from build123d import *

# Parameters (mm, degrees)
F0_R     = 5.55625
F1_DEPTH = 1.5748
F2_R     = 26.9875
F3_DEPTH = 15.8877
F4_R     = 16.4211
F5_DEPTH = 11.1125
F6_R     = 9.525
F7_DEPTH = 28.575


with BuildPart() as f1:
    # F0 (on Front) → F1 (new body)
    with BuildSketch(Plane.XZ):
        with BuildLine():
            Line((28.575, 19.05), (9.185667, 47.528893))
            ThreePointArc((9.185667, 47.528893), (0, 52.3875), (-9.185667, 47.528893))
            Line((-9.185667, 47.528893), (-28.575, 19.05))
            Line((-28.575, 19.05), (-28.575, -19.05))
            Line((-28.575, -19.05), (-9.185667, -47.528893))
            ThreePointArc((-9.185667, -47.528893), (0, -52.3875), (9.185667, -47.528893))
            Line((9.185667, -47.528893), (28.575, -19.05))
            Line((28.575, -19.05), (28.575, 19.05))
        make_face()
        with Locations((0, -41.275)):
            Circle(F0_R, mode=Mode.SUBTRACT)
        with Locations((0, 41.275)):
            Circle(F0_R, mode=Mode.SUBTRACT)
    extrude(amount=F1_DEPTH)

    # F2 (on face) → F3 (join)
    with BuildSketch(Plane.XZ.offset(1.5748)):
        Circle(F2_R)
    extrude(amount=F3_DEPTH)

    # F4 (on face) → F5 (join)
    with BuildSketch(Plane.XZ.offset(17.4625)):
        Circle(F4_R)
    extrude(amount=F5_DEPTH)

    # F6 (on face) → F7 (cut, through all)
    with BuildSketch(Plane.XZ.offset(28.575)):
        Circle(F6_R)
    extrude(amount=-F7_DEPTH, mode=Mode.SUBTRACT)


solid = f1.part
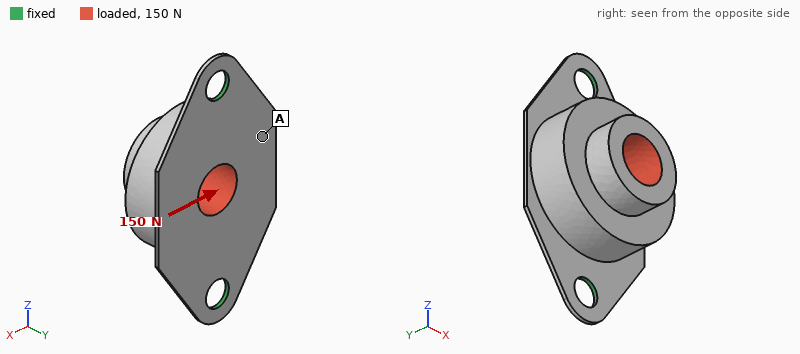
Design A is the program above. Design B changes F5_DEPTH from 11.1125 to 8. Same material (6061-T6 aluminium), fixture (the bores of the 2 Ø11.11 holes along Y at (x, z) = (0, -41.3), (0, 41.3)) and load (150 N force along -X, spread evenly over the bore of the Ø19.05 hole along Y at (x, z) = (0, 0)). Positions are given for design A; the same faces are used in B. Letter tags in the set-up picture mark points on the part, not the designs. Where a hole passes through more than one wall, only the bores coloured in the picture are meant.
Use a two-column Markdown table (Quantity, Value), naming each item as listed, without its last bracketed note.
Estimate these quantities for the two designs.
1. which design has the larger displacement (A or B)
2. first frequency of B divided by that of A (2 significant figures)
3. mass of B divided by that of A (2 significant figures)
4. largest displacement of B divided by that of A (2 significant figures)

| Quantity | Value |
|---|---|
| which design has the larger displacement | A |
| first frequency of B divided by that of A | 1.0 |
| mass of B divided by that of A | 0.96 |
| largest displacement of B divided by that of A | 0.87 |
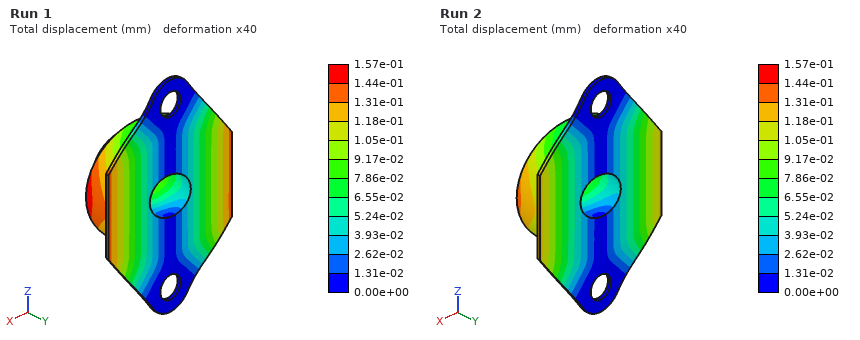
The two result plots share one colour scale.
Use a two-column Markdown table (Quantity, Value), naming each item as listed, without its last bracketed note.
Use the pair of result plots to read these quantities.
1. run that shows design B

| Quantity | Value |
|---|---|
| run that shows design B | Run 2 |
